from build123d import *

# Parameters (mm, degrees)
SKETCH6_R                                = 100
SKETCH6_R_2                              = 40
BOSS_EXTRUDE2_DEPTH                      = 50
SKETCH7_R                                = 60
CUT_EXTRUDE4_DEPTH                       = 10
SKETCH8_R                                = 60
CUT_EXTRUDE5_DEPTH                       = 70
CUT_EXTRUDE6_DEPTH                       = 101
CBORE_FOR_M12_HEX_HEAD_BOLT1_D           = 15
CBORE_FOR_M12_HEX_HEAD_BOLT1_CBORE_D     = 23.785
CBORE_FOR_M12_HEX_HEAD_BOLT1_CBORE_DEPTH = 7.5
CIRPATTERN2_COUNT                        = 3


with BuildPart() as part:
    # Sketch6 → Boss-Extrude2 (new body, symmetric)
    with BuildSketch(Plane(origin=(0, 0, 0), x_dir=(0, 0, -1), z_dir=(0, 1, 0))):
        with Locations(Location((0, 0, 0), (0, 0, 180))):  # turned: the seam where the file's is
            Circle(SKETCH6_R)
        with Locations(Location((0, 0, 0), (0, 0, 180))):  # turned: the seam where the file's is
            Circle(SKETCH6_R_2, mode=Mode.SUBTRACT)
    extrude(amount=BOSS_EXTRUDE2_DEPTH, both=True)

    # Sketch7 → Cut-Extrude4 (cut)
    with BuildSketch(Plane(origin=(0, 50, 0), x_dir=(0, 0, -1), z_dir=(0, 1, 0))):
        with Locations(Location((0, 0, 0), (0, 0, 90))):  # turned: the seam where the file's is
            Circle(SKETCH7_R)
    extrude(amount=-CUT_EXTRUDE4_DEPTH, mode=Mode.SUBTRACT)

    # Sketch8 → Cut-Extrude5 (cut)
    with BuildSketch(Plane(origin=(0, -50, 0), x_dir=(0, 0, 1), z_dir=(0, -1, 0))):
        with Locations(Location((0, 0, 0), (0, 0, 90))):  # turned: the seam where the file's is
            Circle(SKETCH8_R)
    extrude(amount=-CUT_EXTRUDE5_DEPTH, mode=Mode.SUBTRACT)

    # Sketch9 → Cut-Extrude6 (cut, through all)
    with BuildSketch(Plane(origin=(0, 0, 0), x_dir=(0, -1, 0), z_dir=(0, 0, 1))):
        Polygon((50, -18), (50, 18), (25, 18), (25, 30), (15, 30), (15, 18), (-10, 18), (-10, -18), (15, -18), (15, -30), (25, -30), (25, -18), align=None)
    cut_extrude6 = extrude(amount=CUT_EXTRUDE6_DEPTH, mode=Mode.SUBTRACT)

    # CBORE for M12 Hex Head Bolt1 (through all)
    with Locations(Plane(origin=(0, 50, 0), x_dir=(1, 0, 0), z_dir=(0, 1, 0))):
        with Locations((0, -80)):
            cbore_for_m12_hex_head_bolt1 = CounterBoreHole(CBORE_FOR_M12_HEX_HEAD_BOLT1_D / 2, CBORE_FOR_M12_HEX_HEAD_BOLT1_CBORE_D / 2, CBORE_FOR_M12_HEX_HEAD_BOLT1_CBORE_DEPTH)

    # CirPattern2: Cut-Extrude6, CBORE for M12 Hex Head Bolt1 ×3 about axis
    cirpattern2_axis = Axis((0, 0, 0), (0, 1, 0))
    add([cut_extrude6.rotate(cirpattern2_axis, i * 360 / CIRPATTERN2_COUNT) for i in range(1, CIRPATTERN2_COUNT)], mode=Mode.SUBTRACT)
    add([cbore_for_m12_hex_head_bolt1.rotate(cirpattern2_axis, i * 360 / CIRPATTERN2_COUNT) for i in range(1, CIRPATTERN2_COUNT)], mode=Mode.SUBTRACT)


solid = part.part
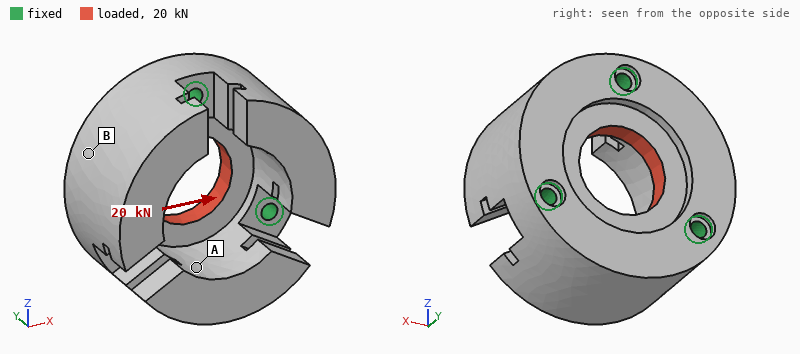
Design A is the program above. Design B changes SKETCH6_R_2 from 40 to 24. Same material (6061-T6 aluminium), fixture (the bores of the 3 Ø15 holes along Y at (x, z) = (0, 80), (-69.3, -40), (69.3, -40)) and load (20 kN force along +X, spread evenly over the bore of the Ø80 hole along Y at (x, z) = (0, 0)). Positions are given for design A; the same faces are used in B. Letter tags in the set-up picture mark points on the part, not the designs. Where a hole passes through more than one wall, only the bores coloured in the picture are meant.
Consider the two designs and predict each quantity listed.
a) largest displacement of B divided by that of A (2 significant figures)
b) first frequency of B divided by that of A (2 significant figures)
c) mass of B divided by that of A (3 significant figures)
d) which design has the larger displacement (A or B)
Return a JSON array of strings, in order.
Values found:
["1.3", "1.0", "1.04", "B"]
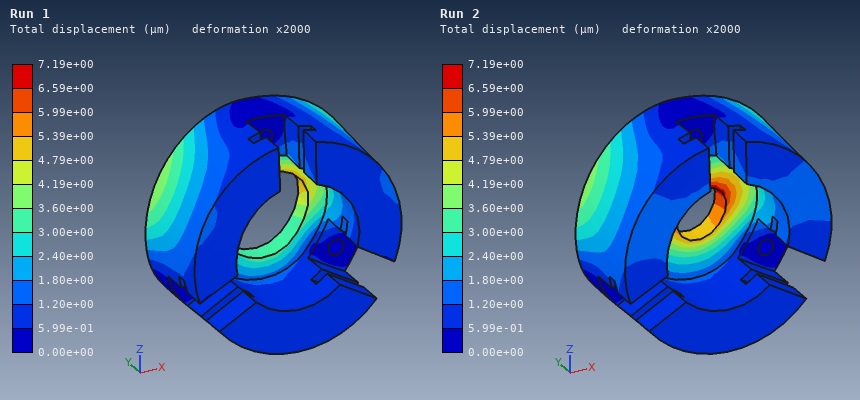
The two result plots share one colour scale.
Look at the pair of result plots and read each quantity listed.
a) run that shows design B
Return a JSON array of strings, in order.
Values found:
["Run 2"]
